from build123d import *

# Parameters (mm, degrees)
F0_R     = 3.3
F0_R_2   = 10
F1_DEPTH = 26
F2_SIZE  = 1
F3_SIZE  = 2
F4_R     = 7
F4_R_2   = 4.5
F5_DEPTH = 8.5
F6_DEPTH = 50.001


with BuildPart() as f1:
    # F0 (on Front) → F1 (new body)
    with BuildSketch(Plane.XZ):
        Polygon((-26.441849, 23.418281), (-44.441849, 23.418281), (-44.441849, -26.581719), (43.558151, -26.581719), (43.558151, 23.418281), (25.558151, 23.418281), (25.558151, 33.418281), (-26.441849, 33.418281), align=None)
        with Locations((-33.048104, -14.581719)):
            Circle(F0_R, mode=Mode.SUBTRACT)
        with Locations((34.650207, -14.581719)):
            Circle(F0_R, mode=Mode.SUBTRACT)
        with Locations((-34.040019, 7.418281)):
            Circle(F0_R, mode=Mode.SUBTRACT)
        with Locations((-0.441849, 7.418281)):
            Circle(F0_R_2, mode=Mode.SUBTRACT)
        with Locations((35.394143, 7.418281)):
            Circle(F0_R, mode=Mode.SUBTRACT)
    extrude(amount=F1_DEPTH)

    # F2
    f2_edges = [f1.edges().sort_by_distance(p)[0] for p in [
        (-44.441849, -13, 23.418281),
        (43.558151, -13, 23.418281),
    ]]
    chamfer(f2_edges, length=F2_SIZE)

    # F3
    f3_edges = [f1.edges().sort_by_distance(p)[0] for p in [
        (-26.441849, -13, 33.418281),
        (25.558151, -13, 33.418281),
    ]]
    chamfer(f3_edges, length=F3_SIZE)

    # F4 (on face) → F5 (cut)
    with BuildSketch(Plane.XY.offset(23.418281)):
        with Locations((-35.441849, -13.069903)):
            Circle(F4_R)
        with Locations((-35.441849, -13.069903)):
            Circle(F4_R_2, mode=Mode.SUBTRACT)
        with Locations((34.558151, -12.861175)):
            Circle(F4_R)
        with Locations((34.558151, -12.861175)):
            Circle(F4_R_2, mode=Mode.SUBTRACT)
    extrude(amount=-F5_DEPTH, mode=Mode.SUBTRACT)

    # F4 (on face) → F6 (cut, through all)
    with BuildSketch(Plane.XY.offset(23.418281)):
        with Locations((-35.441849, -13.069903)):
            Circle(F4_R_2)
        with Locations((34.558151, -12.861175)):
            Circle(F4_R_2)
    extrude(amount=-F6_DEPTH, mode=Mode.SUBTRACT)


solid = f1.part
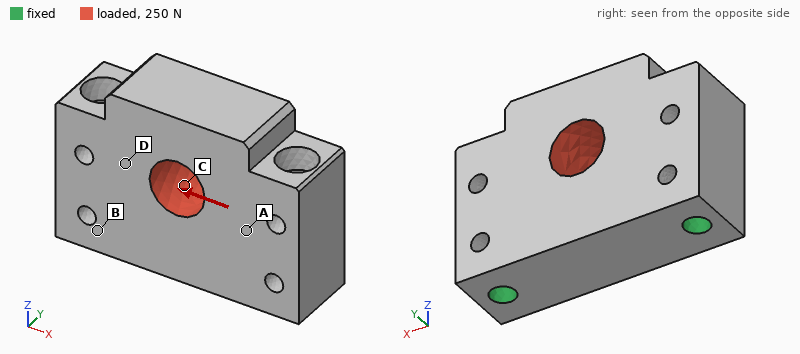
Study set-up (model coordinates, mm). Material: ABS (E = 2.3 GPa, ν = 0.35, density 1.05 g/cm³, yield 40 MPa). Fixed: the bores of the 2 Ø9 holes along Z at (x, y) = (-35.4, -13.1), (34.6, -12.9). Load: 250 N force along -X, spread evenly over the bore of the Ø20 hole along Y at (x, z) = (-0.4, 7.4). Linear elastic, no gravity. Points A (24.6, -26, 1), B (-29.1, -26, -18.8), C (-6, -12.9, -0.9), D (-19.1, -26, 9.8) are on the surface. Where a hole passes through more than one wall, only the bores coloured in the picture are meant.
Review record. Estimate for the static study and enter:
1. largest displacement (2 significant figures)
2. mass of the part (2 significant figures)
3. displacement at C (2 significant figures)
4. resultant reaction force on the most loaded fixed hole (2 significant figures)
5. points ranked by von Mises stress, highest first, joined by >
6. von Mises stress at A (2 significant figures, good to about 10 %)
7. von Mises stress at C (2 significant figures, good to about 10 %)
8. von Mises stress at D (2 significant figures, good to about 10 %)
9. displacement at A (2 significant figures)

3.1 µm
110 g
1.8 µm
130 N
C > D > A > B
0.094 MPa
0.24 MPa
0.18 MPa
0.86 µm
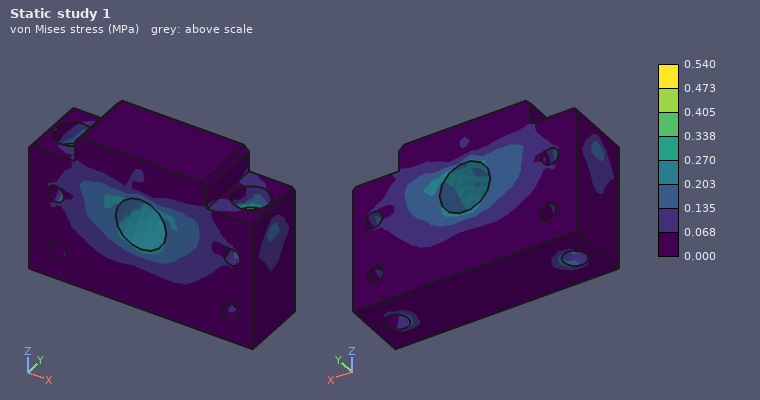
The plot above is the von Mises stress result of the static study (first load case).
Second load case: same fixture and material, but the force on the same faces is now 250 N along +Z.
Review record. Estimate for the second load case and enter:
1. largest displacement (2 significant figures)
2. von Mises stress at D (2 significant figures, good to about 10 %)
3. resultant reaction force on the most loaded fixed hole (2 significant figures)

5.1 µm
0.17 MPa
130 N
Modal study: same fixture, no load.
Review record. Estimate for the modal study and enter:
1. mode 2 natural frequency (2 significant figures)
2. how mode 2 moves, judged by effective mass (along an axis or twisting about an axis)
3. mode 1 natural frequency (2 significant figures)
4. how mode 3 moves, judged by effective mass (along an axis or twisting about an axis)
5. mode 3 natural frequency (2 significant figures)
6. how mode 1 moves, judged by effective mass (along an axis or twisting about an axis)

4500 Hz
along Y
3000 Hz
along Z
5500 Hz
along Y
